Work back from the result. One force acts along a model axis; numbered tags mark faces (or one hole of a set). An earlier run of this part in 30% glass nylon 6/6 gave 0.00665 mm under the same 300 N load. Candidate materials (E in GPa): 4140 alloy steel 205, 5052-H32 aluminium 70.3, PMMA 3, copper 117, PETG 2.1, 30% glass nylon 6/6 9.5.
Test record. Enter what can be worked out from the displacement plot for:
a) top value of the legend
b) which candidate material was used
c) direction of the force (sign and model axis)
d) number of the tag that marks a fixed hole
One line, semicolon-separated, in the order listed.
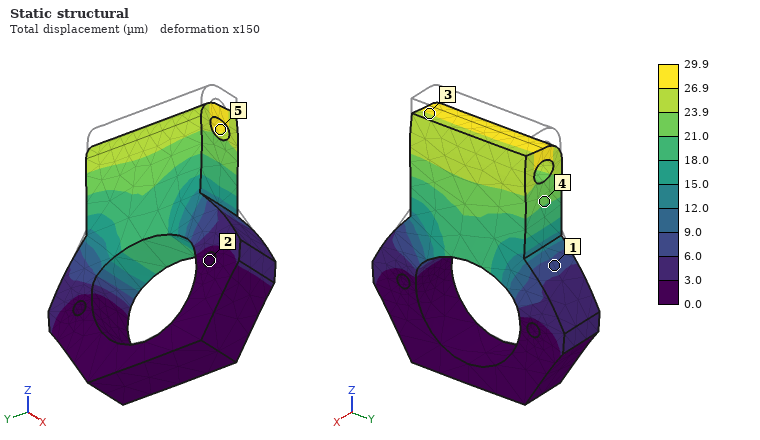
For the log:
29.9 µm; PETG; -Z; 2
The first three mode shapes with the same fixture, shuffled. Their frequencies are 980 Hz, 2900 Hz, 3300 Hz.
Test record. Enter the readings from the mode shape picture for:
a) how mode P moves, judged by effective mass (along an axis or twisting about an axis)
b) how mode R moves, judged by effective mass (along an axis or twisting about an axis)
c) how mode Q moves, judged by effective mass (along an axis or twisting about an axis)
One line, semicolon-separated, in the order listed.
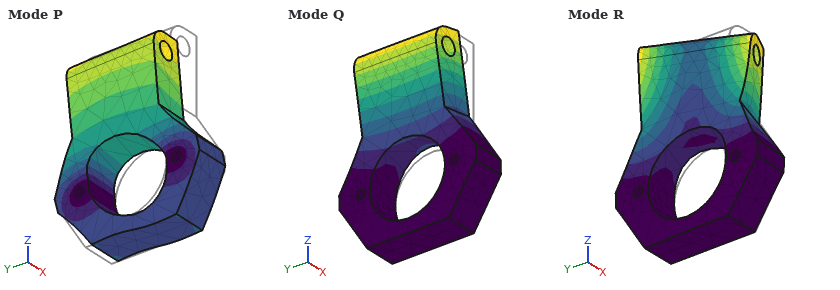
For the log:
along Y; twisting about Z; along X
